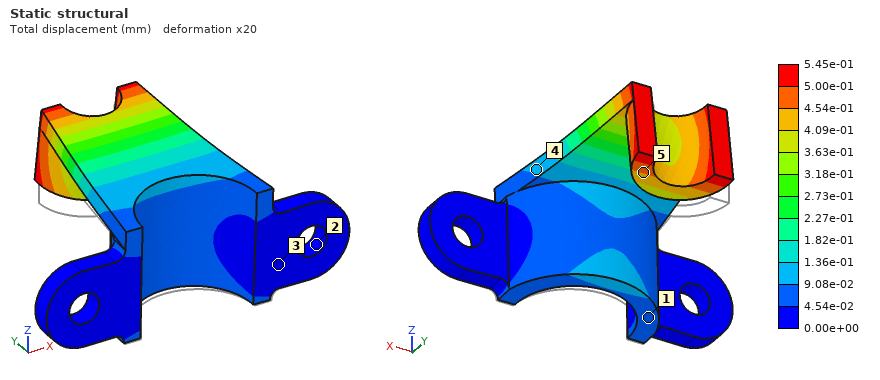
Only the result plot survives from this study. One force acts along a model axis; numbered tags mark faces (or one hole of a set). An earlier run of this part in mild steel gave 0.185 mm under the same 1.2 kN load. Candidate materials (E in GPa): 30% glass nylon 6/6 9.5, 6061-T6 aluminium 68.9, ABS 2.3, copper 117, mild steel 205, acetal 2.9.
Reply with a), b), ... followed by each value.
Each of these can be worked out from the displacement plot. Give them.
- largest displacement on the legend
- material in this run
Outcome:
a) 5.45e-01 mm
b) 6061-T6 aluminium
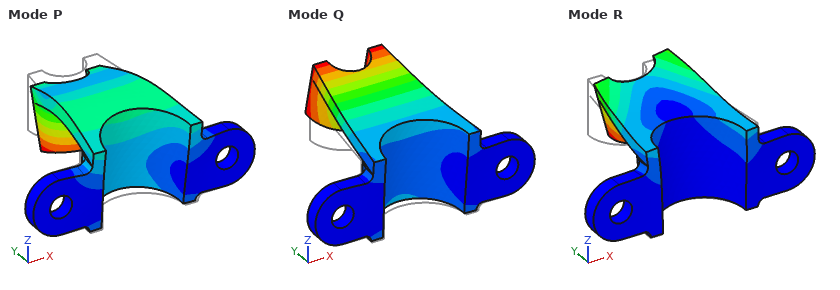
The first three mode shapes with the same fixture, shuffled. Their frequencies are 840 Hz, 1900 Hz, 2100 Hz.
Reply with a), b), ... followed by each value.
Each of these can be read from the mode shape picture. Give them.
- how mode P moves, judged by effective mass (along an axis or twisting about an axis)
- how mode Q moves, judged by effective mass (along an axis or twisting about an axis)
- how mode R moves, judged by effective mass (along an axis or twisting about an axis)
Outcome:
a) along Y
b) along Z
c) along X
